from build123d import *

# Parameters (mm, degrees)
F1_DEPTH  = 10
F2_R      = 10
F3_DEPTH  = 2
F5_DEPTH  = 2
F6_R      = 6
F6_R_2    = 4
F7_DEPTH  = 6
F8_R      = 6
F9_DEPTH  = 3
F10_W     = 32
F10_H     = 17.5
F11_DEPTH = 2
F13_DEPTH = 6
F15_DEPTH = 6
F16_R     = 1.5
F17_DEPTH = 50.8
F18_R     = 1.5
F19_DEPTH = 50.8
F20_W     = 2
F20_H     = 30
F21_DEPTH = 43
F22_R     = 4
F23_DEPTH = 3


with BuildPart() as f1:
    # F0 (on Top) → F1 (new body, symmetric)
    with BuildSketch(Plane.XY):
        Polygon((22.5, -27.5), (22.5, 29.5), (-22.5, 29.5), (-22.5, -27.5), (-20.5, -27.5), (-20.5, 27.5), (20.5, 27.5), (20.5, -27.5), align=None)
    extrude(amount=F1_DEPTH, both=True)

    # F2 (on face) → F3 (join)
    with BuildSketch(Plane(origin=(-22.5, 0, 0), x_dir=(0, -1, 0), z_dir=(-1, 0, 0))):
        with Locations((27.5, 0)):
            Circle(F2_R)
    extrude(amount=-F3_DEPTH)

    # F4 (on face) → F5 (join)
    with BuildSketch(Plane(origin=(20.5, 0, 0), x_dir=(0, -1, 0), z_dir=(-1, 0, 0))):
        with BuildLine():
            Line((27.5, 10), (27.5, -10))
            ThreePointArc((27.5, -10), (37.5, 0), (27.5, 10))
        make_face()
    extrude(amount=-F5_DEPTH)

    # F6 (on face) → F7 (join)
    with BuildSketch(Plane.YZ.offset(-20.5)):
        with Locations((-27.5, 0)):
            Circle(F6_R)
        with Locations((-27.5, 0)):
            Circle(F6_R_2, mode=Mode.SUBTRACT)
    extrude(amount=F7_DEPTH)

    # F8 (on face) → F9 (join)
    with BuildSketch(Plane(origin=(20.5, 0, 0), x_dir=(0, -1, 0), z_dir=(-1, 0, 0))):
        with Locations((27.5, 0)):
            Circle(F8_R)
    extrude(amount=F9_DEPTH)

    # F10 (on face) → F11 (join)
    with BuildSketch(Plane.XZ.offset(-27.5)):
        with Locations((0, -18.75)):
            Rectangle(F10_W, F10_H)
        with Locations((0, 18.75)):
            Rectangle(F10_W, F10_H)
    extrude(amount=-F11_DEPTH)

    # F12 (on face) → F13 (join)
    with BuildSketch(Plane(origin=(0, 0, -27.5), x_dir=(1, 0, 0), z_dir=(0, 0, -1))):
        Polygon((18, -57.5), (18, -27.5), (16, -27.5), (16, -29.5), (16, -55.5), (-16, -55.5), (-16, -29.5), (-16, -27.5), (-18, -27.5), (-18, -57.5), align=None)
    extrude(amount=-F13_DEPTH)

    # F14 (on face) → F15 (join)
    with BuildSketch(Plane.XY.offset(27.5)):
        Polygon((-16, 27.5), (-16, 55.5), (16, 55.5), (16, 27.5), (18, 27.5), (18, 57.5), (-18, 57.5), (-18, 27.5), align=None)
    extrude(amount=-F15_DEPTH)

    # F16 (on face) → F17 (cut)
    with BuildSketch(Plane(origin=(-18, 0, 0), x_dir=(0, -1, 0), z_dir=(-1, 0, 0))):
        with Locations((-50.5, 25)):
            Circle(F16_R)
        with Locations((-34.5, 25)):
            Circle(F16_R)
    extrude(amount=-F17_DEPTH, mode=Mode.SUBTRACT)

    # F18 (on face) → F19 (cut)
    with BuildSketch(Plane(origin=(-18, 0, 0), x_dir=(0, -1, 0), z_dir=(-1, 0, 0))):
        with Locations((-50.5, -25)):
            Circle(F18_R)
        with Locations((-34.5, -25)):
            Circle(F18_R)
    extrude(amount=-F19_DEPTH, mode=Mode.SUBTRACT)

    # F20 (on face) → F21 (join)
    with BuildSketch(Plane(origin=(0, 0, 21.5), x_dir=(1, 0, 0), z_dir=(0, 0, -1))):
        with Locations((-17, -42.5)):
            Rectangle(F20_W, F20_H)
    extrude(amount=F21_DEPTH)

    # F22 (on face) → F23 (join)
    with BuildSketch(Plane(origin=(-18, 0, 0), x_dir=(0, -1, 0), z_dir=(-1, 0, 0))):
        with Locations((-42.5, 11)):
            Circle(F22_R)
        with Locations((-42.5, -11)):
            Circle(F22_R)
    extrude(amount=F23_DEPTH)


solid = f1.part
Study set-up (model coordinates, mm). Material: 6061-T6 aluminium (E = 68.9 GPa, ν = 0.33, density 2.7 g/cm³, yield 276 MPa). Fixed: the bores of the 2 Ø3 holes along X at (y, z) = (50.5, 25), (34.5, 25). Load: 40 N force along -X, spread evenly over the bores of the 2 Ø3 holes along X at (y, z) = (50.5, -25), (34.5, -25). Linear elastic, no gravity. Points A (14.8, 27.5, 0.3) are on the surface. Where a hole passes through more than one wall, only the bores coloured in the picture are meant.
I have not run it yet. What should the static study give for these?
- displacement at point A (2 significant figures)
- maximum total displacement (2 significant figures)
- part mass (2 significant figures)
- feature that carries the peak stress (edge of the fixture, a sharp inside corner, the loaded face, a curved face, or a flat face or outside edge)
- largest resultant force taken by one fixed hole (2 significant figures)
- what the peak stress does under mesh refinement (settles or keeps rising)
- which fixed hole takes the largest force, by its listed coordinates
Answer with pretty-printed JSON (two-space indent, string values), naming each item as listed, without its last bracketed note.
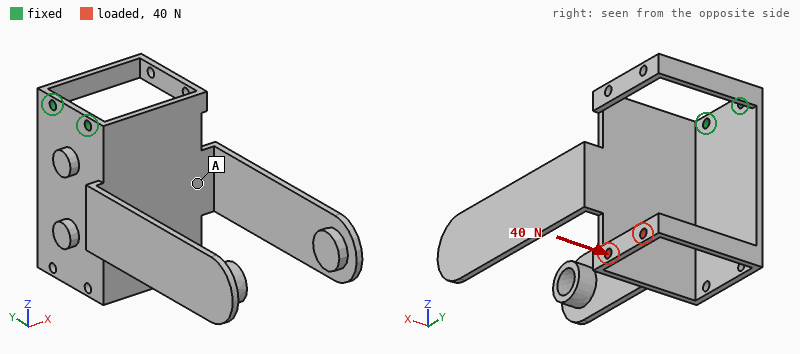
{
  "displacement at point A": "0.26 mm",
  "maximum total displacement": "0.48 mm",
  "part mass": "40 g",
  "feature that carries the peak stress": "edge of the fixture",
  "largest resultant force taken by one fixed hole": "32 N",
  "what the peak stress does under mesh refinement": "keeps rising",
  "which fixed hole takes the largest force, by its listed coordinates": "(34.5, 25)"
}
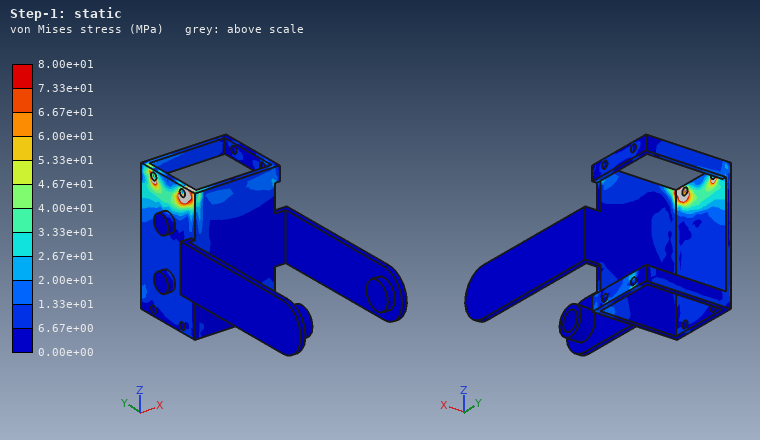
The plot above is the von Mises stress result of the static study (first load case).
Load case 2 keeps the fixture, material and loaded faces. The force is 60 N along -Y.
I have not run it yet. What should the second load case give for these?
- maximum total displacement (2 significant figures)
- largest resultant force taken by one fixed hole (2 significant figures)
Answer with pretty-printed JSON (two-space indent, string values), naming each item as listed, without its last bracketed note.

{
  "maximum total displacement": "1.2 mm",
  "largest resultant force taken by one fixed hole": "190 N"
}
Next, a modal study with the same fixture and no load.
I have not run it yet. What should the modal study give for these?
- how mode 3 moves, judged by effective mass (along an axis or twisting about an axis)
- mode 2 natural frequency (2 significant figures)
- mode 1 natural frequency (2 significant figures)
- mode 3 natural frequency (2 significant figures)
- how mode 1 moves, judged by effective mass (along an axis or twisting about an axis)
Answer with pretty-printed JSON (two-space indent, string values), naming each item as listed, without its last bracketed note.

{
  "how mode 3 moves, judged by effective mass": "along Z",
  "mode 2 natural frequency": "280 Hz",
  "mode 1 natural frequency": "210 Hz",
  "mode 3 natural frequency": "360 Hz",
  "how mode 1 moves, judged by effective mass": "along X"
}
